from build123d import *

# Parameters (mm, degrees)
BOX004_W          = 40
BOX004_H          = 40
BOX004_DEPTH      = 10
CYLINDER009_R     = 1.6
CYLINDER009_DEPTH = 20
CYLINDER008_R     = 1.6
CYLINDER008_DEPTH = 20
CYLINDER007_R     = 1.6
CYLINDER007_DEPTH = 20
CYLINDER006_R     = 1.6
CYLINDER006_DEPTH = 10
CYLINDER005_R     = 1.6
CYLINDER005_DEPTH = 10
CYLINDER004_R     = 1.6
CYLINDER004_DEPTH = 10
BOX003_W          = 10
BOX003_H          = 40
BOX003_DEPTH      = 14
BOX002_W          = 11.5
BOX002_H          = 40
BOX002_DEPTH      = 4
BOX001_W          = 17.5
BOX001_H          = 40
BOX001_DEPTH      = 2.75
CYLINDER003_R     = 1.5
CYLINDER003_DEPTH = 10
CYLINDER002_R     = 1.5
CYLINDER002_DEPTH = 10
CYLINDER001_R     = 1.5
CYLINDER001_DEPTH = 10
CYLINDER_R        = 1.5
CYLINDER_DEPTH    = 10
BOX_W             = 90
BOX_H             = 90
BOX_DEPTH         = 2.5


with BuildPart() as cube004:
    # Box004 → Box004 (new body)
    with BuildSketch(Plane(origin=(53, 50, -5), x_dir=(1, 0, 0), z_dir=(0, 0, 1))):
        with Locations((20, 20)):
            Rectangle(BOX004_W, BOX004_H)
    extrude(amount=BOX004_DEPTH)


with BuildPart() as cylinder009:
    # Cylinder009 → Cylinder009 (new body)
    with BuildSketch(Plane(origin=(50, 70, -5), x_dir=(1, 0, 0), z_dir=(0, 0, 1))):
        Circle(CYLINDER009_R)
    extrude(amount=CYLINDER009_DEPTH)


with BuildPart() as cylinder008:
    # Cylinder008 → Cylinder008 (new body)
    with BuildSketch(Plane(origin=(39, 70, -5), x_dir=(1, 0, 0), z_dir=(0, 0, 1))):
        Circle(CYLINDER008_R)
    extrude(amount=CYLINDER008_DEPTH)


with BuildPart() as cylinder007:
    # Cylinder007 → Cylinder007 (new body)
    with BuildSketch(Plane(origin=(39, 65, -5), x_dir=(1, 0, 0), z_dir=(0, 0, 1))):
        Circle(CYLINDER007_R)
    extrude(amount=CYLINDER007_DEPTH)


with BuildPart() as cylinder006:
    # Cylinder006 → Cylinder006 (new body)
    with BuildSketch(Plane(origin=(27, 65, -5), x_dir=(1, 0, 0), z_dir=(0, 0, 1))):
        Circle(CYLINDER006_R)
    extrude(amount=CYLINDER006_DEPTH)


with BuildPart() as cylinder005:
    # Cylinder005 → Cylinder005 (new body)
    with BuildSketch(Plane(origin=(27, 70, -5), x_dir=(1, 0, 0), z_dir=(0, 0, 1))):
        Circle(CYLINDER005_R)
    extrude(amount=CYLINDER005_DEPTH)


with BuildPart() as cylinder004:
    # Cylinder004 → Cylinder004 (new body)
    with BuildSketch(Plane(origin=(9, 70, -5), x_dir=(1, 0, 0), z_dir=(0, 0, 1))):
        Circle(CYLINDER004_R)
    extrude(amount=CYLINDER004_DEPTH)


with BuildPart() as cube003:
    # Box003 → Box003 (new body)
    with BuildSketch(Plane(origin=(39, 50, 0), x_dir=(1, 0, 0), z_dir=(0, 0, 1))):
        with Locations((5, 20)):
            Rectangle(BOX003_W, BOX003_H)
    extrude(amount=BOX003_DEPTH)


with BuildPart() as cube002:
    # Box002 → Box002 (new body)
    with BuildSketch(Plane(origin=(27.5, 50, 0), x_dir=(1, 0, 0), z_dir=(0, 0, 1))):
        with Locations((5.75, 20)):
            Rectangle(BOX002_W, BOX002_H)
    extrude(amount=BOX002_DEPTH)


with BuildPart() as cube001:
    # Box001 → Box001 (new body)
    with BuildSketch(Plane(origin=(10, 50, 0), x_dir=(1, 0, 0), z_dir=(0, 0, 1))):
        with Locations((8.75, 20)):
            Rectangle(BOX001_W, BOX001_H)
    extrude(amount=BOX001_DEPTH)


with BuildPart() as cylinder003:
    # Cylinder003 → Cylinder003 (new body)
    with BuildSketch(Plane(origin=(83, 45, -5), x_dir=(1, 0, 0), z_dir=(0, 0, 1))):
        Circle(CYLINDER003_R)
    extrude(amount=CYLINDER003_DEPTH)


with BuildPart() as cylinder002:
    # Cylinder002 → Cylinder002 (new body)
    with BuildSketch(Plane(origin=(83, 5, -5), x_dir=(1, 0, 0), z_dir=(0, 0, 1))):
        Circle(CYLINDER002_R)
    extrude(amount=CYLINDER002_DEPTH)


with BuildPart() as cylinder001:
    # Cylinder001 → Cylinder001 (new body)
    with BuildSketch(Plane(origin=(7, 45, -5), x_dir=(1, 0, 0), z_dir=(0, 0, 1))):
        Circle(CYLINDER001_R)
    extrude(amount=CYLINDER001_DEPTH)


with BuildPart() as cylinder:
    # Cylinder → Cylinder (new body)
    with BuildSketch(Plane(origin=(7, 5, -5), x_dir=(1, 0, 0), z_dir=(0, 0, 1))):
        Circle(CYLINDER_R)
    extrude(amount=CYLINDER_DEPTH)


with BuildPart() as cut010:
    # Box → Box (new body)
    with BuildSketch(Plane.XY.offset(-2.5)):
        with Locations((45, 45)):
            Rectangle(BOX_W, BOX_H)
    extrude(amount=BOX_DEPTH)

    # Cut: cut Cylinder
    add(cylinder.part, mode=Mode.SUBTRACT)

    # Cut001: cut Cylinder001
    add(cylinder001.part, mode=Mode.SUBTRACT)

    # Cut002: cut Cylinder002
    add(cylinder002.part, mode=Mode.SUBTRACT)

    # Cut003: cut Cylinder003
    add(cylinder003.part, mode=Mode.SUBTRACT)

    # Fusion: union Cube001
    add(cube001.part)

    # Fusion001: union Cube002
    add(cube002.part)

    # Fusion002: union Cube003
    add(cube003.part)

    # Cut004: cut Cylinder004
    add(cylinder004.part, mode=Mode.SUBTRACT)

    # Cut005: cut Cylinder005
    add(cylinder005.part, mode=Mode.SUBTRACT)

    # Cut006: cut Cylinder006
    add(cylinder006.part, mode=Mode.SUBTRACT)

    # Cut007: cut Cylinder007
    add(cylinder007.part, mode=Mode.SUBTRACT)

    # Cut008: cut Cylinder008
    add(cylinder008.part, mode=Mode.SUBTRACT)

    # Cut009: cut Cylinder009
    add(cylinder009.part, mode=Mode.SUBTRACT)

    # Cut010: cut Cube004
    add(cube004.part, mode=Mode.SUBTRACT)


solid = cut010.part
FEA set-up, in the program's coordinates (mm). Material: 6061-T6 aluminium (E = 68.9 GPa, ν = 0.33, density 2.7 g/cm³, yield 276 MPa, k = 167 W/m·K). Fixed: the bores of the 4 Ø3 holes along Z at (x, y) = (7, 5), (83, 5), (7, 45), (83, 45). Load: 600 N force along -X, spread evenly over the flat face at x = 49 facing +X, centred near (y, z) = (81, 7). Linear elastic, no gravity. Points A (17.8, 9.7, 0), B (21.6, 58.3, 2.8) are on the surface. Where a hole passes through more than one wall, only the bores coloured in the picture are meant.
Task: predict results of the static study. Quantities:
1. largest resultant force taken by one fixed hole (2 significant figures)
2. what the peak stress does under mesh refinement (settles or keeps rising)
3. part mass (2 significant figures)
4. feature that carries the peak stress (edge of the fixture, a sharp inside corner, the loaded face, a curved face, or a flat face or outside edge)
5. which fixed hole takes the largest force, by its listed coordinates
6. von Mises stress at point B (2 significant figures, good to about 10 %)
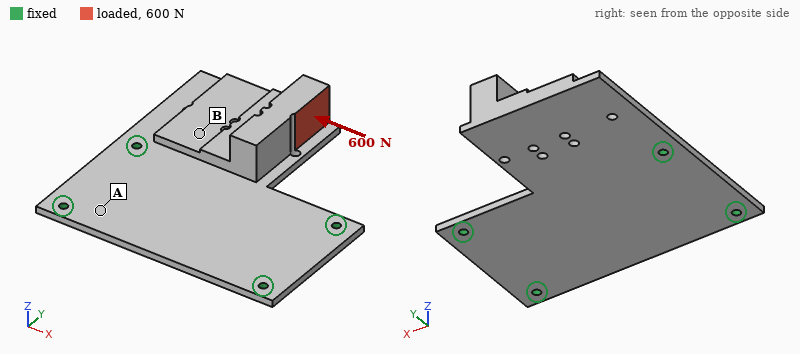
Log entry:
640 N
keeps rising
69 g
edge of the fixture
(7, 45)
15 MPa
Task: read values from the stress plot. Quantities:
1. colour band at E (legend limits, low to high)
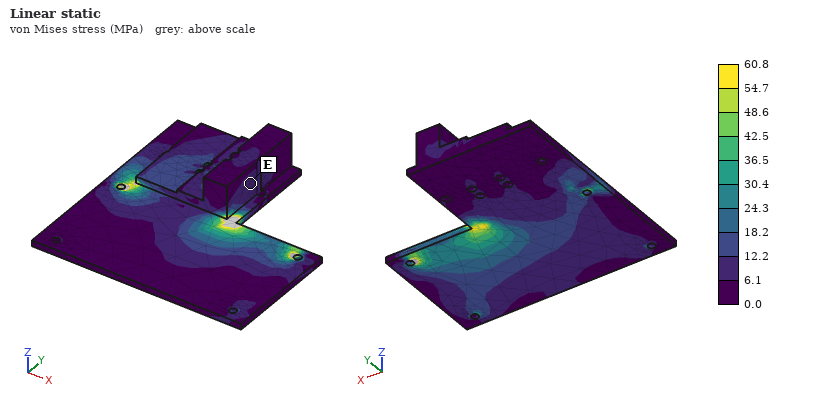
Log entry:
6.1 to 12.2 MPa
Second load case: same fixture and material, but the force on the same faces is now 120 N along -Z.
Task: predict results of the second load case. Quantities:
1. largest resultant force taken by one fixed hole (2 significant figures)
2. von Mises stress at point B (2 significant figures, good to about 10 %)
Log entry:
95 N
16 MPa
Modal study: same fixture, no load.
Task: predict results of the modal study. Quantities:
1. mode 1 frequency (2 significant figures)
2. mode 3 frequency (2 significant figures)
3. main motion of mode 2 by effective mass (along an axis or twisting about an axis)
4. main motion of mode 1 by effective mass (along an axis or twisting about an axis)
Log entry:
530 Hz
2700 Hz
along Z
along Z
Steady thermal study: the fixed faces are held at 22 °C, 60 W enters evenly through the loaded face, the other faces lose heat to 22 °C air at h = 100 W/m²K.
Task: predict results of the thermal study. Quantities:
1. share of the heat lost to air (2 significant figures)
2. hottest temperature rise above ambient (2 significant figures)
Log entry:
56 %
72 K
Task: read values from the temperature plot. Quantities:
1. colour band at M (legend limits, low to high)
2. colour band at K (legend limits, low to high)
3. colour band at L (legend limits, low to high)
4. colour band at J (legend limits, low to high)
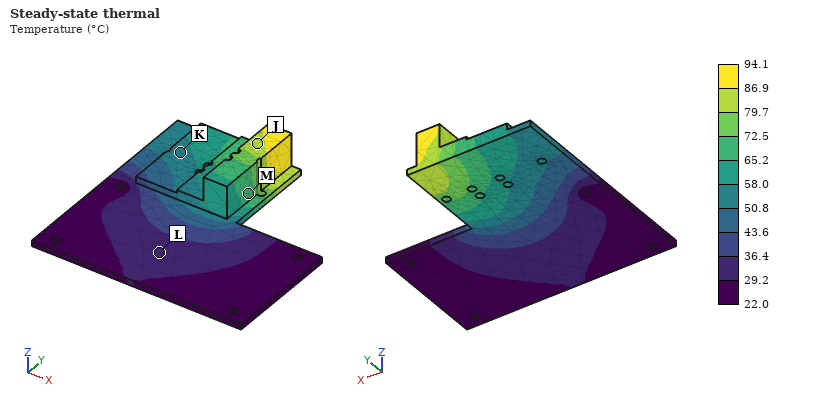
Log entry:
65.2 to 72.5 °C
50.8 to 58.0 °C
29.2 to 36.4 °C
79.7 to 86.9 °C
